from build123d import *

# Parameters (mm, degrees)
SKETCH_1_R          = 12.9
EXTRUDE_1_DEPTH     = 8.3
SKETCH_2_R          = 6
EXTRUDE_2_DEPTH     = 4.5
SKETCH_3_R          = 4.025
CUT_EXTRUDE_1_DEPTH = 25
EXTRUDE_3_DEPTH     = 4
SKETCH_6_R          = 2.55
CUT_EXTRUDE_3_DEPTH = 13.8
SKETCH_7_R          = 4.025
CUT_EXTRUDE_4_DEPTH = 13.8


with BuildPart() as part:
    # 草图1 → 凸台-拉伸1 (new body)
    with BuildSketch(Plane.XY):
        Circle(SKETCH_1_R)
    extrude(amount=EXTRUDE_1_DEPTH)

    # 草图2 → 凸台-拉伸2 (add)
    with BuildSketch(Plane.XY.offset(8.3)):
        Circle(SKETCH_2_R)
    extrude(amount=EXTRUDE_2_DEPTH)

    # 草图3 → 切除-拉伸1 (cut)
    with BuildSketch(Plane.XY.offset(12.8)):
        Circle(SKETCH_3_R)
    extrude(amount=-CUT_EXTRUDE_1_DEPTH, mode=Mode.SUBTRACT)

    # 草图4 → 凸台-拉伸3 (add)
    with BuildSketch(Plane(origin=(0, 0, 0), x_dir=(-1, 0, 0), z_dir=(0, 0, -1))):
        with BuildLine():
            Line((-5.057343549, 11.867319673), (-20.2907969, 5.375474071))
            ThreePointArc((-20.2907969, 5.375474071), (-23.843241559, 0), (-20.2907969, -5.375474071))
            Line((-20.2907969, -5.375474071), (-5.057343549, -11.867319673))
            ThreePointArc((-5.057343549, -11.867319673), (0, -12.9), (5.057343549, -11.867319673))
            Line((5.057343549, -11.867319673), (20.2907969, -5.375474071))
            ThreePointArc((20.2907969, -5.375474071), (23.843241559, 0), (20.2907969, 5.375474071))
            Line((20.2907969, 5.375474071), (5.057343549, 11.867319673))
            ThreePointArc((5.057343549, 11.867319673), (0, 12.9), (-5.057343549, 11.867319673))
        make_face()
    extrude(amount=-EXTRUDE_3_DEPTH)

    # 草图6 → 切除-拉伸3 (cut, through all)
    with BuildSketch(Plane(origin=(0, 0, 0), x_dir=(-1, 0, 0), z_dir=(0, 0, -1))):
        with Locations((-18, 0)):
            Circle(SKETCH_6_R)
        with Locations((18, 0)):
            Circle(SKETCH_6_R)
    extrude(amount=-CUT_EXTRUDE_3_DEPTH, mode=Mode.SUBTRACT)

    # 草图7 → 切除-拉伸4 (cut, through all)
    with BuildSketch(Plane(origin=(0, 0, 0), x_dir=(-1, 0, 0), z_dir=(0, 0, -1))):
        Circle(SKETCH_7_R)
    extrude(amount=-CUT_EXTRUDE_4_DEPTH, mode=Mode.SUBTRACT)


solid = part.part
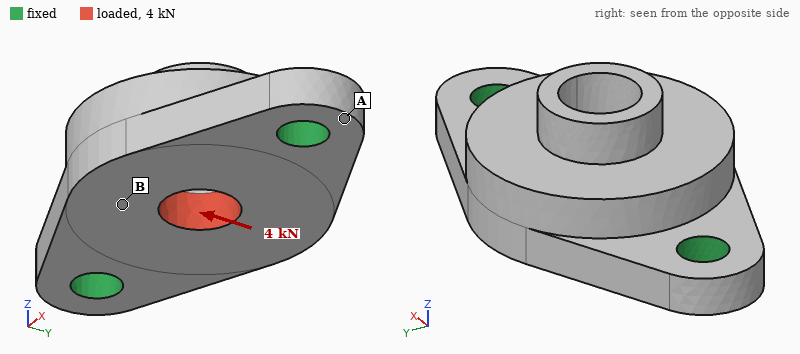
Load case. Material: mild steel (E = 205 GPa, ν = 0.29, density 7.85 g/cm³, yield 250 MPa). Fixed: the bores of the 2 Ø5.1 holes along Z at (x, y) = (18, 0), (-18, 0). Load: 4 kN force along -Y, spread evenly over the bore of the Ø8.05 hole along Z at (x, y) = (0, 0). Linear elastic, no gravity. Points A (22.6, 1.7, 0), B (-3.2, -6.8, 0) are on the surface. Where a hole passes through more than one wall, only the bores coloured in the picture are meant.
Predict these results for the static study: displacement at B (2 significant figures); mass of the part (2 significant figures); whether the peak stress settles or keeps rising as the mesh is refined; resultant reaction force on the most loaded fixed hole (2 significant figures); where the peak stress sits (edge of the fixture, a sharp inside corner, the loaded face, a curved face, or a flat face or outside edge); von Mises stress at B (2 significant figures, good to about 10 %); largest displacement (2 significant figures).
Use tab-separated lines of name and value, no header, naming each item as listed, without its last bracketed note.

displacement at B	5.5 µm
mass of the part	41 g
whether the peak stress settles or keeps rising as the mesh is refined	keeps rising
resultant reaction force on the most loaded fixed hole	2.0 kN
where the peak stress sits	edge of the fixture
von Mises stress at B	37 MPa
largest displacement	6.4 µm
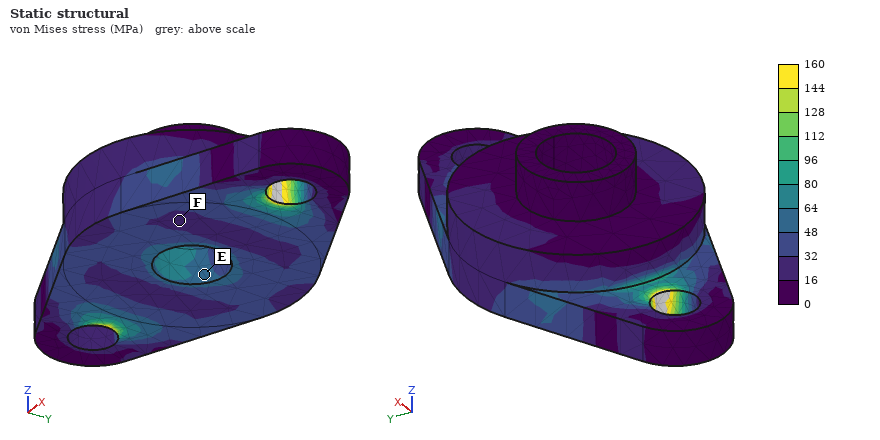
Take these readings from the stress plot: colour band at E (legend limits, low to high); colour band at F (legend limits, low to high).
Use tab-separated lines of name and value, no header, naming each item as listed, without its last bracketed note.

colour band at E	48 to 64 MPa
colour band at F	16 to 32 MPa
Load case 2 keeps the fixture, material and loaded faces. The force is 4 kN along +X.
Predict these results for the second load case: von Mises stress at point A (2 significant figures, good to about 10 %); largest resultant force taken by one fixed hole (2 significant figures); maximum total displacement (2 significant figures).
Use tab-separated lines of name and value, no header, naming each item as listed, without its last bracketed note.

von Mises stress at point A	11 MPa
largest resultant force taken by one fixed hole	2.0 kN
maximum total displacement	2.9 µm
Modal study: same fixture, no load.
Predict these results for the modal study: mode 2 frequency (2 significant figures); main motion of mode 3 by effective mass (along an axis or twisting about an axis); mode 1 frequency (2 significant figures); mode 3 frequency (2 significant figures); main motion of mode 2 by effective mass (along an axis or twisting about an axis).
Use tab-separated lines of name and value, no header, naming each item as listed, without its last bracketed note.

mode 2 frequency	17 kHz
main motion of mode 3 by effective mass	along Y
mode 1 frequency	11 kHz
mode 3 frequency	28 kHz
main motion of mode 2 by effective mass	along Z
